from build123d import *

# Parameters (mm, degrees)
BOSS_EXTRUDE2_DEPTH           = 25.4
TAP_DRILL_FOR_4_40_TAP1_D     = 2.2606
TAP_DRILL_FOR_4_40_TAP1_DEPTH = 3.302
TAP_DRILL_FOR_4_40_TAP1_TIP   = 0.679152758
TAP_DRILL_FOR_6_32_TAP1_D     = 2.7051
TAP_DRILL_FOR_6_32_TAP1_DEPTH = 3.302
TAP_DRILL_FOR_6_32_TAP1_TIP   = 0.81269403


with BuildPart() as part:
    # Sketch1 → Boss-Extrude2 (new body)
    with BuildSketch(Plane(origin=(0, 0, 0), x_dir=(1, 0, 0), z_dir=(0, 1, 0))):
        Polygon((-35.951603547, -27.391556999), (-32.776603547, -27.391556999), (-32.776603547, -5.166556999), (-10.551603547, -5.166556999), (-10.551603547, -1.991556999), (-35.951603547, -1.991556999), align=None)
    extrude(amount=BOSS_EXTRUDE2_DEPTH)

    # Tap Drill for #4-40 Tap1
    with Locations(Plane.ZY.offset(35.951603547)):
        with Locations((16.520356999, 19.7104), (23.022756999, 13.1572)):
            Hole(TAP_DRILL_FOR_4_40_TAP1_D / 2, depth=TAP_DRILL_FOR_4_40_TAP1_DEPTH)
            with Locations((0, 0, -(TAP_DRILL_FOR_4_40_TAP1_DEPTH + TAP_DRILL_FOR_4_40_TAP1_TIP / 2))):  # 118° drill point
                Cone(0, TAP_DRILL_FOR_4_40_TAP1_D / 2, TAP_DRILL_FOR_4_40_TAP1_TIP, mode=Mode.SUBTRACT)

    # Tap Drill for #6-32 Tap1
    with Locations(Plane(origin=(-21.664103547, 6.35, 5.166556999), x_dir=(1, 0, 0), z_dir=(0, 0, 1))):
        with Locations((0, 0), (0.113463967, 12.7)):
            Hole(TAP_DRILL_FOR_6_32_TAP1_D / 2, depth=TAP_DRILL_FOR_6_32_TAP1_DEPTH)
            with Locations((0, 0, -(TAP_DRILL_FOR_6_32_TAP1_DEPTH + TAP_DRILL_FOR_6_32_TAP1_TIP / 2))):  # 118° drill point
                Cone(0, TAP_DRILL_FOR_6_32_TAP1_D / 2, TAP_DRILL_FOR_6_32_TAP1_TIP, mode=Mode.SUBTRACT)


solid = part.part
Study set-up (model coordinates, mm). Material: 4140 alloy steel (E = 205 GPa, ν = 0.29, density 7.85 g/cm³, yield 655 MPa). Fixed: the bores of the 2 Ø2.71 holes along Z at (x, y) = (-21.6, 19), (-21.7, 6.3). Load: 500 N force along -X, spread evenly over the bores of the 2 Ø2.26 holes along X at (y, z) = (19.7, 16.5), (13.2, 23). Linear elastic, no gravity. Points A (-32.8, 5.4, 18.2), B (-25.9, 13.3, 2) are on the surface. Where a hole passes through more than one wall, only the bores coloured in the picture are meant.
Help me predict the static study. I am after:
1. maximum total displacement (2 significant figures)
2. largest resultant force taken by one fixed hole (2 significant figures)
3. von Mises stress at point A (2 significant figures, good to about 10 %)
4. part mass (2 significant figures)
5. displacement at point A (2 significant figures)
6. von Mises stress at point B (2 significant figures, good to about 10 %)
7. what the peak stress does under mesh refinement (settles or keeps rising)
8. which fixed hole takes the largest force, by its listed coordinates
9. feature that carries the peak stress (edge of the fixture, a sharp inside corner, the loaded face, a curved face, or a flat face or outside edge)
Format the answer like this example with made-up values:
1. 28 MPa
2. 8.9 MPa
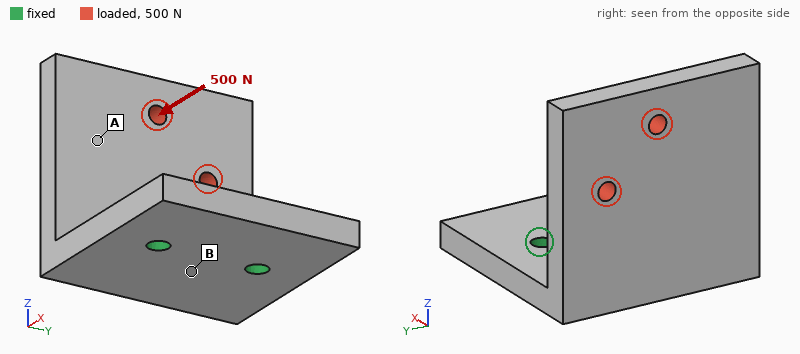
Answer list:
1. 0.26 mm
2. 390 N
3. 46 MPa
4. 30 g
5. 0.14 mm
6. 150 MPa
7. keeps rising
8. (-21.6, 19)
9. edge of the fixture
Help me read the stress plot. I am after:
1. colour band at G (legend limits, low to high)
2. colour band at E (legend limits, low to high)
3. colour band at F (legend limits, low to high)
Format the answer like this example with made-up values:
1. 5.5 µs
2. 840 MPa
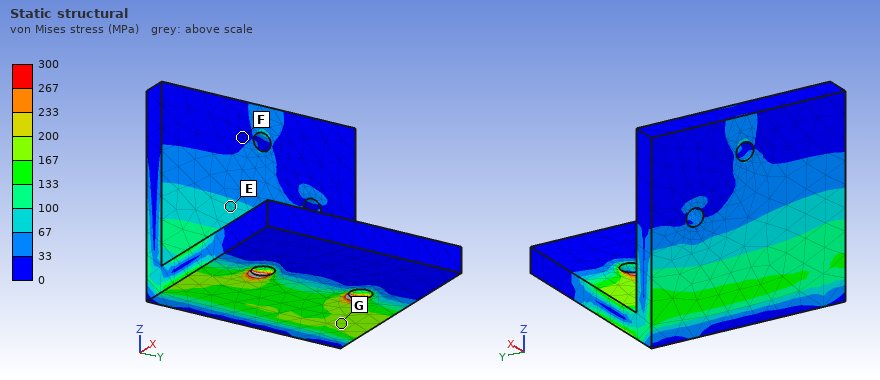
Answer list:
1. 167 to 200 MPa
2. 67 to 100 MPa
3. 0 to 33 MPa
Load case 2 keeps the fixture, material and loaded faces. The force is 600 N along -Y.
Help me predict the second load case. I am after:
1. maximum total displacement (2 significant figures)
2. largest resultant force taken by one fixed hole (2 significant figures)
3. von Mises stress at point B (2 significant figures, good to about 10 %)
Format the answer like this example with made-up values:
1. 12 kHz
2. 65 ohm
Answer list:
1. 80 µm
2. 840 N
3. 73 MPa
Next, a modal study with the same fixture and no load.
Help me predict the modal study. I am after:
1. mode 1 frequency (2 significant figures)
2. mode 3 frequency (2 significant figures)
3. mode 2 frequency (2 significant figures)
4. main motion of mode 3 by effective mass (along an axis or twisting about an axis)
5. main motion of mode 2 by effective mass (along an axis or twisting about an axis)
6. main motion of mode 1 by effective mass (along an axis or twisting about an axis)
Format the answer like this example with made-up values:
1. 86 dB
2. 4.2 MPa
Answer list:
1. 2500 Hz
2. 8100 Hz
3. 4700 Hz
4. along Z
5. along Y
6. along X
